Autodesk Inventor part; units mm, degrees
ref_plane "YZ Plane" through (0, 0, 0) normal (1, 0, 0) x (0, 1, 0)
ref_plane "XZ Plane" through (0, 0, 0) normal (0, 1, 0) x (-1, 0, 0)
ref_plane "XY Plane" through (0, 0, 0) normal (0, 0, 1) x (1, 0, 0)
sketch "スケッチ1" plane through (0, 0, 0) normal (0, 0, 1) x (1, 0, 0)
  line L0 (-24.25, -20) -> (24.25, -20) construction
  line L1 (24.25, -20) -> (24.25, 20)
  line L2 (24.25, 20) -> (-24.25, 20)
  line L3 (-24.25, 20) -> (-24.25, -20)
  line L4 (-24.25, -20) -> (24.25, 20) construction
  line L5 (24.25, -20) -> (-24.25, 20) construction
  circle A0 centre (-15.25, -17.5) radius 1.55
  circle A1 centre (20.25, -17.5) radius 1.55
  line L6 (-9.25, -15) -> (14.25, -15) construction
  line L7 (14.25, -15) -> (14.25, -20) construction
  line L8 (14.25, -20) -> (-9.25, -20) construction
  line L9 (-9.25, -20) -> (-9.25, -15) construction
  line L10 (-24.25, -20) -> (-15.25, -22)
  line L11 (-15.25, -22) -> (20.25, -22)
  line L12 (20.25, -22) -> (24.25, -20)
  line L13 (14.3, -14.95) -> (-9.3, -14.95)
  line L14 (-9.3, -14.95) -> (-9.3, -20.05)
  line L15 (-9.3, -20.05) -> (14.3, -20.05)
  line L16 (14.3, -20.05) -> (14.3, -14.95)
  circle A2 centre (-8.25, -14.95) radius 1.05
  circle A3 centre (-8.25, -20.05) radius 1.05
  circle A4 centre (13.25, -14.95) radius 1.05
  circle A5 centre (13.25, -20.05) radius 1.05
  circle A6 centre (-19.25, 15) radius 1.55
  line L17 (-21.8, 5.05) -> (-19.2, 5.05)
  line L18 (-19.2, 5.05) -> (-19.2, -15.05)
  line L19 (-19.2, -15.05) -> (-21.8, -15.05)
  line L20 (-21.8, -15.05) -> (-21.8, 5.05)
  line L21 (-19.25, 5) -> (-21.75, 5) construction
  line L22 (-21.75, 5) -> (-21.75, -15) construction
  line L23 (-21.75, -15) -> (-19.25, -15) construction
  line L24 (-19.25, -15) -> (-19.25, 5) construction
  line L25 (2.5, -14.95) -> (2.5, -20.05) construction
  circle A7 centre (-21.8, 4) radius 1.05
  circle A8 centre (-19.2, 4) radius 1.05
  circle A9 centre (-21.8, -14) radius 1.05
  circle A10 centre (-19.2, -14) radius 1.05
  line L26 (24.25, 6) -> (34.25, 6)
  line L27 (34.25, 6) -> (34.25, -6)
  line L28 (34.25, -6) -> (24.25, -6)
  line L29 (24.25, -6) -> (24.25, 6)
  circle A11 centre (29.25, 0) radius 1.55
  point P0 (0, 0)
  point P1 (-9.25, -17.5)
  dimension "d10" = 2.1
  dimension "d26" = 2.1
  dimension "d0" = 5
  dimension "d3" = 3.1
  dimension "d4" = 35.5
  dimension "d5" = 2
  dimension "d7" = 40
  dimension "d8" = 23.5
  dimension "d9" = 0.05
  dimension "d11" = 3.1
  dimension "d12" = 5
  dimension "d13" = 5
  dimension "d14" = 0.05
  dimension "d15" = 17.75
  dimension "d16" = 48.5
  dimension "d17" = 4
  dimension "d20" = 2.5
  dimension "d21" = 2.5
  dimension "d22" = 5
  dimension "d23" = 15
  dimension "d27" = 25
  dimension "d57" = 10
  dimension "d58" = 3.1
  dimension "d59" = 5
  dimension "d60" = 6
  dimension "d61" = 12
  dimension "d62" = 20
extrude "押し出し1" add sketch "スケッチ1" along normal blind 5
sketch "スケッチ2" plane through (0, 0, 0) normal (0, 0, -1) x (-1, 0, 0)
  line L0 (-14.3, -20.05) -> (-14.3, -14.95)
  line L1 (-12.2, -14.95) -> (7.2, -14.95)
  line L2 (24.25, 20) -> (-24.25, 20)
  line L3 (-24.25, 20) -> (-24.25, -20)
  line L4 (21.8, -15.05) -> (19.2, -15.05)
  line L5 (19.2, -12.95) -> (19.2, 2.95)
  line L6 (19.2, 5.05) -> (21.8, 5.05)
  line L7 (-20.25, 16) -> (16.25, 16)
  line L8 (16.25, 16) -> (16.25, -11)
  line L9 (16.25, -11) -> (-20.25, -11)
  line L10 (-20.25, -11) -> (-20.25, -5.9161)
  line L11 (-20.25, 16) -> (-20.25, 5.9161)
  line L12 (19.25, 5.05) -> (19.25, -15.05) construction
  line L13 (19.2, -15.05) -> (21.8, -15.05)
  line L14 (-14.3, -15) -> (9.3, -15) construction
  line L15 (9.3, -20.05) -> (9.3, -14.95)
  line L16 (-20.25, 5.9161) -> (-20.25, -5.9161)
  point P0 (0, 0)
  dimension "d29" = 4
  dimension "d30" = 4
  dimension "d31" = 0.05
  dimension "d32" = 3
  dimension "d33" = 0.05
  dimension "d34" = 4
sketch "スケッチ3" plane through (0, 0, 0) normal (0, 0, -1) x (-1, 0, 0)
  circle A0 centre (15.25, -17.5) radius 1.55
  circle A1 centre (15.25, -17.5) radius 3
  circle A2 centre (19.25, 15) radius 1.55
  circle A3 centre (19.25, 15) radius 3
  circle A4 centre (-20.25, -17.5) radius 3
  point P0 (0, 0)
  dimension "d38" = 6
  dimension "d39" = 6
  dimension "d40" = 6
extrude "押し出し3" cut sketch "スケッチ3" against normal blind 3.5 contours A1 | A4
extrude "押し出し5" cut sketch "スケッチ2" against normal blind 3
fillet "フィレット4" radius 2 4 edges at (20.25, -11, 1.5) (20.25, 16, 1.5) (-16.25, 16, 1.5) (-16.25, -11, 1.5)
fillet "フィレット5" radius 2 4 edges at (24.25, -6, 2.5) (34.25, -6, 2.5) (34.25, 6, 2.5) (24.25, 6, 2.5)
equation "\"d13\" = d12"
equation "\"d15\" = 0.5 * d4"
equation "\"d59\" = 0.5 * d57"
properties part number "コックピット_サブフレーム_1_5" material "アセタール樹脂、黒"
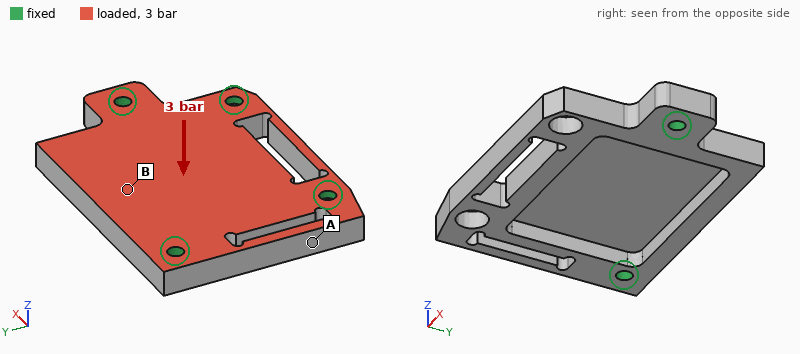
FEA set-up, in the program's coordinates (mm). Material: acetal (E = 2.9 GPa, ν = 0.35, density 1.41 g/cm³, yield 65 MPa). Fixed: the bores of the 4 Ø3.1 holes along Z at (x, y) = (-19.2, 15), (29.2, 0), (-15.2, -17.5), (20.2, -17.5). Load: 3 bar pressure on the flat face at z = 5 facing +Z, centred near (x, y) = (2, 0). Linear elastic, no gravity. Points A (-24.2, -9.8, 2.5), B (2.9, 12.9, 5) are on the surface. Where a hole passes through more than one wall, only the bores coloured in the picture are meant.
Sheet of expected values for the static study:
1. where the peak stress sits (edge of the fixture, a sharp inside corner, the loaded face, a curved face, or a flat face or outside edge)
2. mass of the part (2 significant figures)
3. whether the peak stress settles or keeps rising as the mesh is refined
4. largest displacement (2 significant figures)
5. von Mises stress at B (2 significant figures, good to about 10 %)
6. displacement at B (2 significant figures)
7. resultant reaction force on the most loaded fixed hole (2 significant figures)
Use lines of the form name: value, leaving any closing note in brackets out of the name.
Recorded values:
where the peak stress sits: edge of the fixture
mass of the part: 9.2 g
whether the peak stress settles or keeps rising as the mesh is refined: keeps rising
largest displacement: 0.66 mm
von Mises stress at B: 15 MPa
displacement at B: 0.59 mm
resultant reaction force on the most loaded fixed hole: 230 N
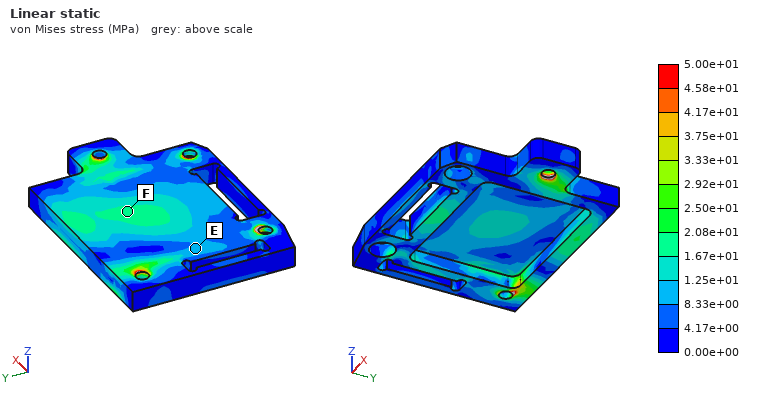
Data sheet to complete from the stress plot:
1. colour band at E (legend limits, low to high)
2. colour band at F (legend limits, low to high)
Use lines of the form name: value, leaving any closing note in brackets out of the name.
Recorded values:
colour band at E: 8.33e+00 to 1.25e+01 MPa
colour band at F: 1.67e+01 to 2.08e+01 MPa
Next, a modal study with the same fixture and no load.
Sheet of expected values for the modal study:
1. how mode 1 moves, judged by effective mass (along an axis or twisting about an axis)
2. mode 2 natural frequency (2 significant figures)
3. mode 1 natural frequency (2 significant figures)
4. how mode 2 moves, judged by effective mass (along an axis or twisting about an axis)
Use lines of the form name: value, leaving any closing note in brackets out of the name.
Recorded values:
how mode 1 moves, judged by effective mass: along Z
mode 2 natural frequency: 2700 Hz
mode 1 natural frequency: 2000 Hz
how mode 2 moves, judged by effective mass: along Z
